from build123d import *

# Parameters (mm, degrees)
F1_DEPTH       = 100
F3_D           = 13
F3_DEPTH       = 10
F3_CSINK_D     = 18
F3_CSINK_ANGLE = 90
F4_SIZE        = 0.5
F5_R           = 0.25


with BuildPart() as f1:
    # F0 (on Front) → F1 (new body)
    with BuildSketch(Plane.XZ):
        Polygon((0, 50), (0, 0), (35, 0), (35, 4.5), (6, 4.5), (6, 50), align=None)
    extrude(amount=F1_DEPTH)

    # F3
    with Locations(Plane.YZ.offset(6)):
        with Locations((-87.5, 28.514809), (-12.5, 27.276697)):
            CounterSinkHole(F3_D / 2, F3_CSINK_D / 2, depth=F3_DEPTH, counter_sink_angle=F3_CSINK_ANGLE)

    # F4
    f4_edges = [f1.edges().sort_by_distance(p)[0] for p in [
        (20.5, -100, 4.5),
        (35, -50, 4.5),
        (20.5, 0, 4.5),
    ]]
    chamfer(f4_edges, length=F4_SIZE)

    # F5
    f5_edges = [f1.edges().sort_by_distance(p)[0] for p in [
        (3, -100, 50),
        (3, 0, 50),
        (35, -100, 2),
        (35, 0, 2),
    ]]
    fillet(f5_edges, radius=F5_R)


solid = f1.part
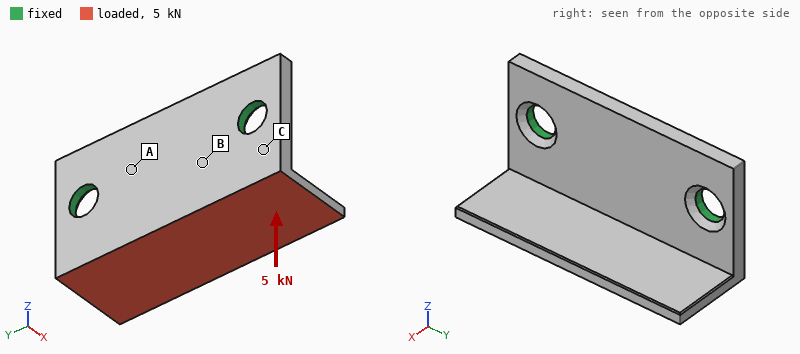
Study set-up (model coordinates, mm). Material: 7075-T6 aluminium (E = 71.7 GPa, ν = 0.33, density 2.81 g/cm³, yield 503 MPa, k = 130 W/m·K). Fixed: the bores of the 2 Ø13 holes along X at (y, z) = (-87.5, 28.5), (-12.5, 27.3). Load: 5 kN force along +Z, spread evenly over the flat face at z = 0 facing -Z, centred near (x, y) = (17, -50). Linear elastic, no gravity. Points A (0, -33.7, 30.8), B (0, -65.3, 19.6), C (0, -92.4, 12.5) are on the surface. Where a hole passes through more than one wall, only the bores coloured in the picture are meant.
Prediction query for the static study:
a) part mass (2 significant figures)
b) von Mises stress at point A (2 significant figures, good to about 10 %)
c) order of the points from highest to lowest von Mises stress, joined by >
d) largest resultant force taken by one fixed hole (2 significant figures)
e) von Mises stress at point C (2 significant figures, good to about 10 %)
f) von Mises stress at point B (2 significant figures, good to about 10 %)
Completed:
120 g
35 MPa
C > B > A
2.5 kN
120 MPa
76 MPa
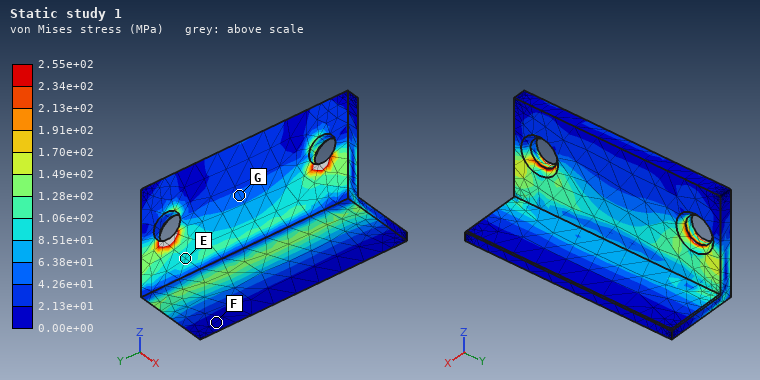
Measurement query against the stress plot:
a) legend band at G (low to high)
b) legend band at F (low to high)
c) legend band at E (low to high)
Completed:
4.26e+01 to 6.38e+01 MPa
0.00e+00 to 2.13e+01 MPa
8.51e+01 to 1.06e+02 MPa
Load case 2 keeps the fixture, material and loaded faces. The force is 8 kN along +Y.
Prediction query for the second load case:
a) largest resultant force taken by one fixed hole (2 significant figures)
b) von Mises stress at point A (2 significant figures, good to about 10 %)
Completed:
5.1 kN
12 MPa
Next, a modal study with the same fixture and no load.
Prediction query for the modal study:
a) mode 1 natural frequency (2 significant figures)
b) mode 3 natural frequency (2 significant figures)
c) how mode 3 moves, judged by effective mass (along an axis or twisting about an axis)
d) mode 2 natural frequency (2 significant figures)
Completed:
2000 Hz
4700 Hz
along X
3100 Hz
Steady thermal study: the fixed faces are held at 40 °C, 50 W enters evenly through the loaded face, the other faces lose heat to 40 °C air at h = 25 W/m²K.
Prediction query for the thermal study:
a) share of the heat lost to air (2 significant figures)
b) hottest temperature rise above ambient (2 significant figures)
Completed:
8.4 %
29 K
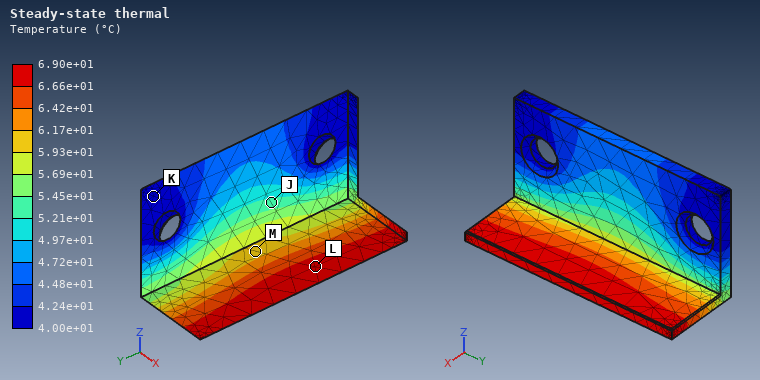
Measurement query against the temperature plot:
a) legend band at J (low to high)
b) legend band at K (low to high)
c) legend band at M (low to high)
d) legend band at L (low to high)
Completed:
5.21e+01 to 5.45e+01 °C
4.00e+01 to 4.24e+01 °C
5.93e+01 to 6.17e+01 °C
6.66e+01 to 6.90e+01 °C
